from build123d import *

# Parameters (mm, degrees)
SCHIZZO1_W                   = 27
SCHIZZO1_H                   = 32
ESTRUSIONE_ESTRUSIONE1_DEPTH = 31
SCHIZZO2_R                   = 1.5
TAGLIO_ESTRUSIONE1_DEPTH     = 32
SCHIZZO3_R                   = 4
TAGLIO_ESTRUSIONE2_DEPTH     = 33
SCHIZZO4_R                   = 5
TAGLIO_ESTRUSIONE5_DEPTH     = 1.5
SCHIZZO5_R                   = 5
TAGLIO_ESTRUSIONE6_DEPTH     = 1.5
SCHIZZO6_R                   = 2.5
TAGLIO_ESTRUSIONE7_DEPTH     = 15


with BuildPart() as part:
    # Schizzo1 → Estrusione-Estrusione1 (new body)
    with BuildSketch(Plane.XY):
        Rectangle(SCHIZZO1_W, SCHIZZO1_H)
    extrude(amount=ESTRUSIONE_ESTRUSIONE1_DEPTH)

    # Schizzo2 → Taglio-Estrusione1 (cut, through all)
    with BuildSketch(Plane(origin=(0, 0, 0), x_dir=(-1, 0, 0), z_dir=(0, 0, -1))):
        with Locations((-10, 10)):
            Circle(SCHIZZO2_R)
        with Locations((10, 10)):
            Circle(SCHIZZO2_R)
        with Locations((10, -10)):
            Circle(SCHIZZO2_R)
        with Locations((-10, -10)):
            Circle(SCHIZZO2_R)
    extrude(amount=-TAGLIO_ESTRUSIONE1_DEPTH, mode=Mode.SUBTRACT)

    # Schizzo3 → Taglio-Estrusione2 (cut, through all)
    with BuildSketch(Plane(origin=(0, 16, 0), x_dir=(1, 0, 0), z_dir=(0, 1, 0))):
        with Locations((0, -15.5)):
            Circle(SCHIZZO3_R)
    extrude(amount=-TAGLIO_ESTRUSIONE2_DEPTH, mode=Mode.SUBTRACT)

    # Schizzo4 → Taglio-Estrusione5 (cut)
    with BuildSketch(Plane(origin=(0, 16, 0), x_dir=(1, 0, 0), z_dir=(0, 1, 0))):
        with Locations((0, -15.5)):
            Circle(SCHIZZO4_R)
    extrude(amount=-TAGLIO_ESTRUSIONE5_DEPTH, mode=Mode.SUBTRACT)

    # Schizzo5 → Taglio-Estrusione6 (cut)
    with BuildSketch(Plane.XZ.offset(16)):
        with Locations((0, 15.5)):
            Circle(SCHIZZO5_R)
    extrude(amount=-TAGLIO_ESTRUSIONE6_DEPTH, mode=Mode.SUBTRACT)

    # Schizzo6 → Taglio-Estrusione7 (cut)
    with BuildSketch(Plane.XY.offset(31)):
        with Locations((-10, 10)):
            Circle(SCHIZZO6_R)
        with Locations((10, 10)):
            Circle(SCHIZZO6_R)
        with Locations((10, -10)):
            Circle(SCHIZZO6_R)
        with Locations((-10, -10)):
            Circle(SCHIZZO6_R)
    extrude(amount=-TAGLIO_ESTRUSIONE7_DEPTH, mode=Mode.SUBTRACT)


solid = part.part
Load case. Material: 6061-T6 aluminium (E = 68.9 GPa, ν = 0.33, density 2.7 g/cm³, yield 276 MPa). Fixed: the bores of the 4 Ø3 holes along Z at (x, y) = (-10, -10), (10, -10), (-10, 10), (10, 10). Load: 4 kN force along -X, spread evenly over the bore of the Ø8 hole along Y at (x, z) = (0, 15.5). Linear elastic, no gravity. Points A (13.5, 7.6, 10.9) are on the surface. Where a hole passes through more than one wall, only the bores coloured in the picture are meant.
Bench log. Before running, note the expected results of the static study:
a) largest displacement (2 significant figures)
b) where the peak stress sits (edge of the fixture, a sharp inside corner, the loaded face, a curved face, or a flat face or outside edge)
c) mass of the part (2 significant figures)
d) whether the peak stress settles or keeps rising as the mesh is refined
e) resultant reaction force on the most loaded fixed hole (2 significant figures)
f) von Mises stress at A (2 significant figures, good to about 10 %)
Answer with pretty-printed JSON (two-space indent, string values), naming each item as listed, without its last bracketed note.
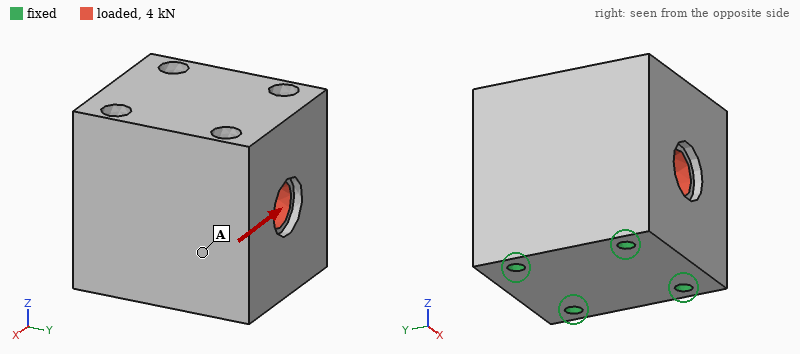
{
  "largest displacement": "2.4 µm",
  "where the peak stress sits": "edge of the fixture",
  "mass of the part": "63 g",
  "whether the peak stress settles or keeps rising as the mesh is refined": "keeps rising",
  "resultant reaction force on the most loaded fixed hole": "1.1 kN",
  "von Mises stress at A": "5.8 MPa"
}
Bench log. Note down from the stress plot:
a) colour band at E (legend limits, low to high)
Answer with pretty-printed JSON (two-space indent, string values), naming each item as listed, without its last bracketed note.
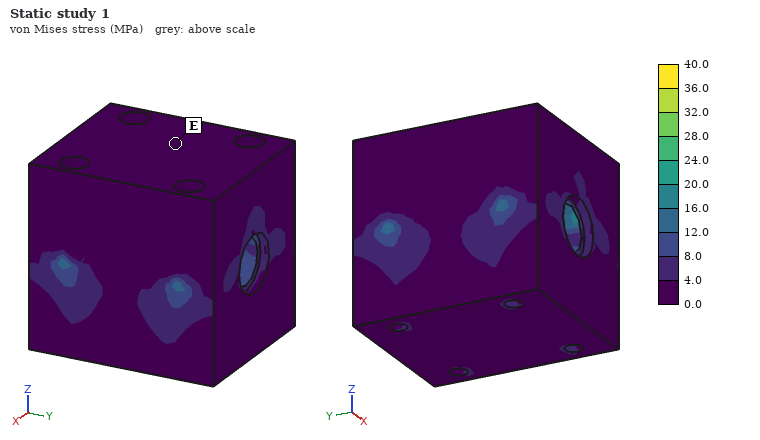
{
  "colour band at E": "0.0 to 4.0 MPa"
}
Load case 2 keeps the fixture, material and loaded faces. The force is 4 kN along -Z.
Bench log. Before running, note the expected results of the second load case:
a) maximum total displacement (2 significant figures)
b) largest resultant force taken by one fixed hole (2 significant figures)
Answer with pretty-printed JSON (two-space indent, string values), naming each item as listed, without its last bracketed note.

{
  "maximum total displacement": "1.8 µm",
  "largest resultant force taken by one fixed hole": "1.0 kN"
}
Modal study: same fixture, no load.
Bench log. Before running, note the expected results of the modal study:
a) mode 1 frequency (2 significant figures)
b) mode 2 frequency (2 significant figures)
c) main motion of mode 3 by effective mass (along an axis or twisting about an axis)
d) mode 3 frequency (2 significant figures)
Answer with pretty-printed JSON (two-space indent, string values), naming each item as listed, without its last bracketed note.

{
  "mode 1 frequency": "25 kHz",
  "mode 2 frequency": "26 kHz",
  "main motion of mode 3 by effective mass": "twisting about Z",
  "mode 3 frequency": "33 kHz"
}
